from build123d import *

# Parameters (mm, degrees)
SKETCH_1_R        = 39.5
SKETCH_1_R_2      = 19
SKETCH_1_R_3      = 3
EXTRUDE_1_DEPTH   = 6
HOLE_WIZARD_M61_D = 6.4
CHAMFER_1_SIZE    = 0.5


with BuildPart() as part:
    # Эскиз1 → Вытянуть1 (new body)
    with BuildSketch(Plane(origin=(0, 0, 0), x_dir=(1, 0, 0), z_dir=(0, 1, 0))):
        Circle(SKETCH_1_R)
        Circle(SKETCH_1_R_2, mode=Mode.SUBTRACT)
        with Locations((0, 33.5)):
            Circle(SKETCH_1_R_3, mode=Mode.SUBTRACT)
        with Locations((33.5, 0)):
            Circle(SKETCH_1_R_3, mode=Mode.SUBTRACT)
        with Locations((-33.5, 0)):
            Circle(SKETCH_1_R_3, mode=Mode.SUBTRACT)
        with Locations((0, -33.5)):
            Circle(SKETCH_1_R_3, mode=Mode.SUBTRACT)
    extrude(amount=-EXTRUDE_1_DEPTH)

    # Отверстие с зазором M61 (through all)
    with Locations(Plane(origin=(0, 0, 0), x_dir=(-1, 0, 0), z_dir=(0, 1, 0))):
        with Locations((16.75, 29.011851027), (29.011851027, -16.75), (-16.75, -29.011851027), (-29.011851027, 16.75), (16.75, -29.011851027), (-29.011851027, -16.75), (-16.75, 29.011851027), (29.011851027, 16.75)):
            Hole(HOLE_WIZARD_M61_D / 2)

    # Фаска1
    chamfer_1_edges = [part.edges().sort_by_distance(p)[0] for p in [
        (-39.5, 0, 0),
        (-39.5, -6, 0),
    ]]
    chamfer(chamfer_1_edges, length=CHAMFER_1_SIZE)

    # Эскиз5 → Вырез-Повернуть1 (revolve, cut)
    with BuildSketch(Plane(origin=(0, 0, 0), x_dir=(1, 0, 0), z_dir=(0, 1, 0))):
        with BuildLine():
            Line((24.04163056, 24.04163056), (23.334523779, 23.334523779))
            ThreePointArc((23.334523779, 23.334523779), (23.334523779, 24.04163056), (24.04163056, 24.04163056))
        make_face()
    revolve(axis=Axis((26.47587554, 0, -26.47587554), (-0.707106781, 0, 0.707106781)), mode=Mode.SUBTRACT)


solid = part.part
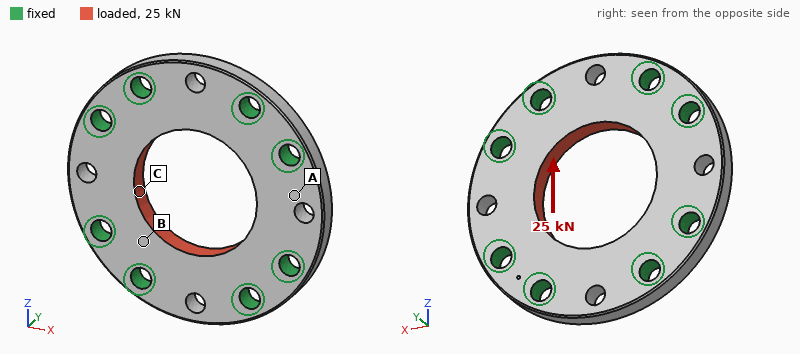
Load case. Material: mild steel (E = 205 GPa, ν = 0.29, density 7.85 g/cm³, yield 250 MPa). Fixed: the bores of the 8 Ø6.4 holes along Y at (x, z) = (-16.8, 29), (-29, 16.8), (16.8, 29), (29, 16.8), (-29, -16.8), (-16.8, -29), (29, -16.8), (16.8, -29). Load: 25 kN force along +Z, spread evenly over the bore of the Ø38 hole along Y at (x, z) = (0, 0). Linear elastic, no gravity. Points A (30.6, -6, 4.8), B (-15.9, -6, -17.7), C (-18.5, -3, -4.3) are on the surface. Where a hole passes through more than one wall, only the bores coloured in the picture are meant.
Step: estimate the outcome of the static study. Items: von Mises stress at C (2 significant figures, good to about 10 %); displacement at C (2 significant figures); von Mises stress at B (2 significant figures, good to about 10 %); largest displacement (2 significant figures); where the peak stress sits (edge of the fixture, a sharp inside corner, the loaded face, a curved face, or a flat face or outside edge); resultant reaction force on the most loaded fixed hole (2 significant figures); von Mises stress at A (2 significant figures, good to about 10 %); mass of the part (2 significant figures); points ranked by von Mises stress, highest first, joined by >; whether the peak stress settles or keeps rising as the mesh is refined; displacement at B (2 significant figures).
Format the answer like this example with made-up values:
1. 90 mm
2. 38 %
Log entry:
1. 60 MPa
2. 3.2 µm
3. 42 MPa
4. 5.1 µm
5. edge of the fixture
6. 4.3 kN
7. 14 MPa
8. 160 g
9. C > B > A
10. keeps rising
11. 1.9 µm
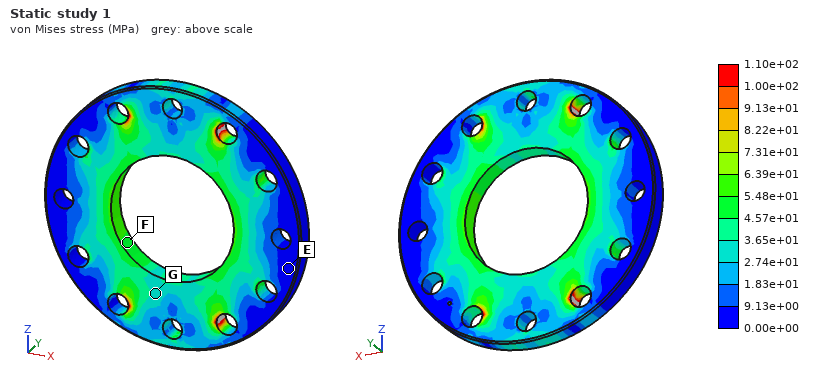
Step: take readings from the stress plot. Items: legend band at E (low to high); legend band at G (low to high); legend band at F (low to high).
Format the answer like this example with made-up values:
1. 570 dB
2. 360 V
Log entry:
1. 0.00e+00 to 9.13e+00 MPa
2. 2.74e+01 to 3.65e+01 MPa
3. 4.57e+01 to 5.48e+01 MPa
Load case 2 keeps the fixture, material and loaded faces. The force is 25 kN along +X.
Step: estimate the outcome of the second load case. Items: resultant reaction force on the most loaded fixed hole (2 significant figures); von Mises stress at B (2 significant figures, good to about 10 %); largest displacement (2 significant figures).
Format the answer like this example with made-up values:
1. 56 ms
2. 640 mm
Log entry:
1. 4.3 kN
2. 38 MPa
3. 5.1 µm
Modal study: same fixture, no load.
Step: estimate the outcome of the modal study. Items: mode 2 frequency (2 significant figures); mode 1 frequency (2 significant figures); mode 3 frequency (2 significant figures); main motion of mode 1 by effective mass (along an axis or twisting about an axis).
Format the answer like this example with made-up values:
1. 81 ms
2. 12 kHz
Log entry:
1. 26 kHz
2. 24 kHz
3. 26 kHz
4. along Y
